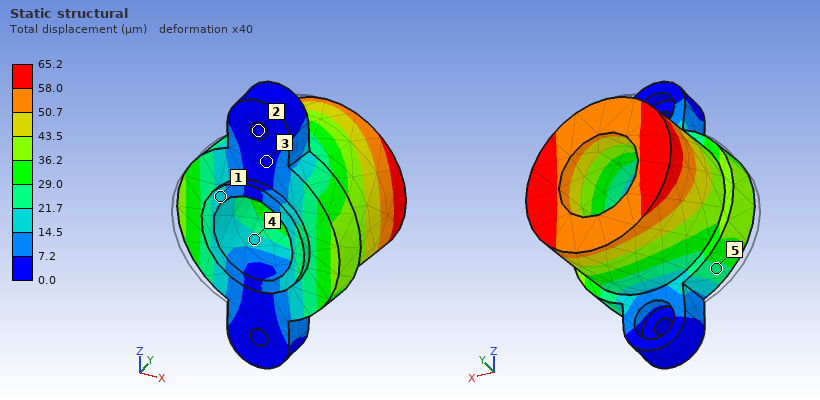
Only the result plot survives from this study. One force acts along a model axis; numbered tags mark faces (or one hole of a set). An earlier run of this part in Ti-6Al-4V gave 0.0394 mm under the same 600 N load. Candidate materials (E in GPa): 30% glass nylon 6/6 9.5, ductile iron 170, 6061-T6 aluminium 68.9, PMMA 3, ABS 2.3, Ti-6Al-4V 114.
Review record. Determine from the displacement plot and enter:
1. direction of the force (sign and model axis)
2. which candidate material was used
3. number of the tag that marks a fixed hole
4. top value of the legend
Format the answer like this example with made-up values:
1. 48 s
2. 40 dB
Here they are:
1. +X
2. 6061-T6 aluminium
3. 2
4. 65.2 µm
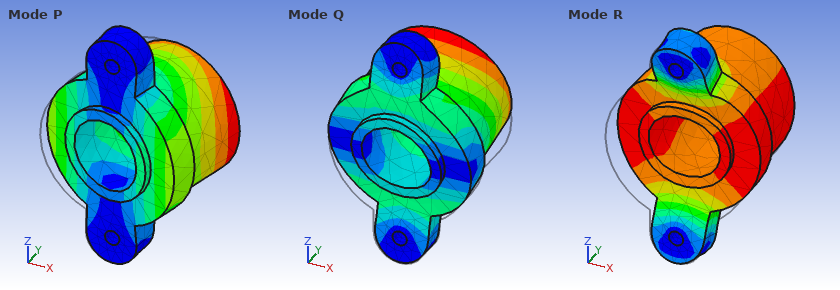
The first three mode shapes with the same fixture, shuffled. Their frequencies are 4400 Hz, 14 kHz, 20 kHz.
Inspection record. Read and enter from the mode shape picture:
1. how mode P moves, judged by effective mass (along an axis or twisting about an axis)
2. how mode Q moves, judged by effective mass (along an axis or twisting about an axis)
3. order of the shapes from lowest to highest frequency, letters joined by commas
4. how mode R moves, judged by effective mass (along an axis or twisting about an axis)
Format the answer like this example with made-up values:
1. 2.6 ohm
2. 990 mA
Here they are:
1. along X
2. along Z
3. P, R, Q
4. along Y
